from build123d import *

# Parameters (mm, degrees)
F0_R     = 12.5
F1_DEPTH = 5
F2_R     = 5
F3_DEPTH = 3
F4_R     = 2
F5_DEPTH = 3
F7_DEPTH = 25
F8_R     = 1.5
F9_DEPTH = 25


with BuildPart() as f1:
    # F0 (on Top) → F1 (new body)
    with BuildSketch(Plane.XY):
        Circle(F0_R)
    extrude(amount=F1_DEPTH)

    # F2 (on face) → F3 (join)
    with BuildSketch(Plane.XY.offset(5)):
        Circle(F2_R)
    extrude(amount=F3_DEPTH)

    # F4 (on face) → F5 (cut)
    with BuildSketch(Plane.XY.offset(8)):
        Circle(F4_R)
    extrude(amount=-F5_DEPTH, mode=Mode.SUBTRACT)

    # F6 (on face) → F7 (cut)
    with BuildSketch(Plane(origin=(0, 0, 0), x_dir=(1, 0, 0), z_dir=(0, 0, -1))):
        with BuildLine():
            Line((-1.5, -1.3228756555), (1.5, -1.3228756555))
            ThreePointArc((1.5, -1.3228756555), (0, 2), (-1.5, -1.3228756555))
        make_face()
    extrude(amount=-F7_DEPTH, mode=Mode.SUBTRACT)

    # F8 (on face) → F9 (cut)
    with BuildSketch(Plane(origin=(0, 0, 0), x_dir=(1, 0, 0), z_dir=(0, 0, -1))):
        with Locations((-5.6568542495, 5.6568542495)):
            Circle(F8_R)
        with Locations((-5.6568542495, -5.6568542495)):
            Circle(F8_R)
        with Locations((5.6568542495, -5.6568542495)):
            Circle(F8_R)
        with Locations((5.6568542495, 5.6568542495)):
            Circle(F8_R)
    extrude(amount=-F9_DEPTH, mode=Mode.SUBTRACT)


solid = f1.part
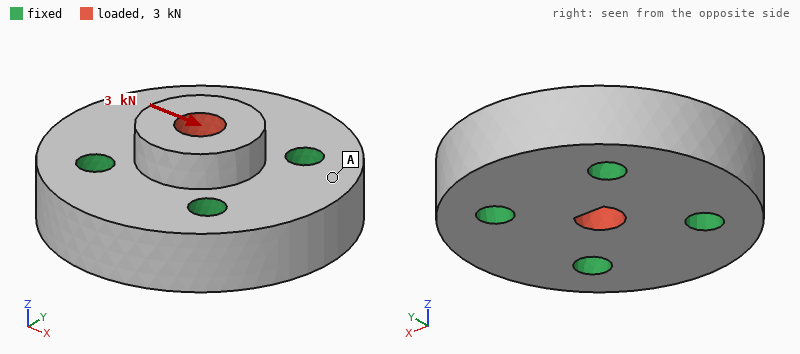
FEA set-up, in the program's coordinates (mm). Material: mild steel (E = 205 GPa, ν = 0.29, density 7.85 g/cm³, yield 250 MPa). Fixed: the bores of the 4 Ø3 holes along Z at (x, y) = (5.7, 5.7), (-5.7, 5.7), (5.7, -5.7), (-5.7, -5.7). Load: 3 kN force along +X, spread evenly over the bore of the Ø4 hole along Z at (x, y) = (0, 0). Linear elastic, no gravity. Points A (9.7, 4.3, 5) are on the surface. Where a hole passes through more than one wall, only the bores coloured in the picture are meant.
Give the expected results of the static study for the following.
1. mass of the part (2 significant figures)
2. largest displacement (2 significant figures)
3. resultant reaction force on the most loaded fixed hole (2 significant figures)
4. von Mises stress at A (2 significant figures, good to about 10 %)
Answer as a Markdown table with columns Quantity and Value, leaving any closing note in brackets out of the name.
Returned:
| Quantity | Value |
|---|---|
| mass of the part | 19 g |
| largest displacement | 2.3 µm |
| resultant reaction force on the most loaded fixed hole | 910 N |
| von Mises stress at A | 8.7 MPa |
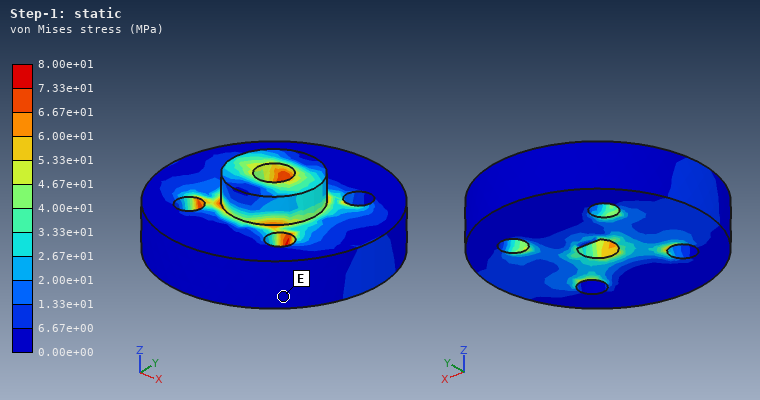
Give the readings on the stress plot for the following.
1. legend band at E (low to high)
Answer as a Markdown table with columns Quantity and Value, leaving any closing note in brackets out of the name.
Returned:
| Quantity | Value |
|---|---|
| legend band at E | 0.00e+00 to 6.67e+00 MPa |
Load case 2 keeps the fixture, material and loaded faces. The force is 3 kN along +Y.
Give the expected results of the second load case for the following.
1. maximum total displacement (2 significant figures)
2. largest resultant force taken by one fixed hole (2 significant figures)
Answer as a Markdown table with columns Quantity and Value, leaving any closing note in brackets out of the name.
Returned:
| Quantity | Value |
|---|---|
| maximum total displacement | 2.3 µm |
| largest resultant force taken by one fixed hole | 890 N |
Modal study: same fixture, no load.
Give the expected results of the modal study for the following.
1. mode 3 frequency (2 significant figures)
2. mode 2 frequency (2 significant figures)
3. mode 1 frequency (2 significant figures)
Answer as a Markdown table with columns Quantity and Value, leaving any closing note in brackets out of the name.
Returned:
| Quantity | Value |
|---|---|
| mode 3 frequency | 79 kHz |
| mode 2 frequency | 79 kHz |
| mode 1 frequency | 77 kHz |
